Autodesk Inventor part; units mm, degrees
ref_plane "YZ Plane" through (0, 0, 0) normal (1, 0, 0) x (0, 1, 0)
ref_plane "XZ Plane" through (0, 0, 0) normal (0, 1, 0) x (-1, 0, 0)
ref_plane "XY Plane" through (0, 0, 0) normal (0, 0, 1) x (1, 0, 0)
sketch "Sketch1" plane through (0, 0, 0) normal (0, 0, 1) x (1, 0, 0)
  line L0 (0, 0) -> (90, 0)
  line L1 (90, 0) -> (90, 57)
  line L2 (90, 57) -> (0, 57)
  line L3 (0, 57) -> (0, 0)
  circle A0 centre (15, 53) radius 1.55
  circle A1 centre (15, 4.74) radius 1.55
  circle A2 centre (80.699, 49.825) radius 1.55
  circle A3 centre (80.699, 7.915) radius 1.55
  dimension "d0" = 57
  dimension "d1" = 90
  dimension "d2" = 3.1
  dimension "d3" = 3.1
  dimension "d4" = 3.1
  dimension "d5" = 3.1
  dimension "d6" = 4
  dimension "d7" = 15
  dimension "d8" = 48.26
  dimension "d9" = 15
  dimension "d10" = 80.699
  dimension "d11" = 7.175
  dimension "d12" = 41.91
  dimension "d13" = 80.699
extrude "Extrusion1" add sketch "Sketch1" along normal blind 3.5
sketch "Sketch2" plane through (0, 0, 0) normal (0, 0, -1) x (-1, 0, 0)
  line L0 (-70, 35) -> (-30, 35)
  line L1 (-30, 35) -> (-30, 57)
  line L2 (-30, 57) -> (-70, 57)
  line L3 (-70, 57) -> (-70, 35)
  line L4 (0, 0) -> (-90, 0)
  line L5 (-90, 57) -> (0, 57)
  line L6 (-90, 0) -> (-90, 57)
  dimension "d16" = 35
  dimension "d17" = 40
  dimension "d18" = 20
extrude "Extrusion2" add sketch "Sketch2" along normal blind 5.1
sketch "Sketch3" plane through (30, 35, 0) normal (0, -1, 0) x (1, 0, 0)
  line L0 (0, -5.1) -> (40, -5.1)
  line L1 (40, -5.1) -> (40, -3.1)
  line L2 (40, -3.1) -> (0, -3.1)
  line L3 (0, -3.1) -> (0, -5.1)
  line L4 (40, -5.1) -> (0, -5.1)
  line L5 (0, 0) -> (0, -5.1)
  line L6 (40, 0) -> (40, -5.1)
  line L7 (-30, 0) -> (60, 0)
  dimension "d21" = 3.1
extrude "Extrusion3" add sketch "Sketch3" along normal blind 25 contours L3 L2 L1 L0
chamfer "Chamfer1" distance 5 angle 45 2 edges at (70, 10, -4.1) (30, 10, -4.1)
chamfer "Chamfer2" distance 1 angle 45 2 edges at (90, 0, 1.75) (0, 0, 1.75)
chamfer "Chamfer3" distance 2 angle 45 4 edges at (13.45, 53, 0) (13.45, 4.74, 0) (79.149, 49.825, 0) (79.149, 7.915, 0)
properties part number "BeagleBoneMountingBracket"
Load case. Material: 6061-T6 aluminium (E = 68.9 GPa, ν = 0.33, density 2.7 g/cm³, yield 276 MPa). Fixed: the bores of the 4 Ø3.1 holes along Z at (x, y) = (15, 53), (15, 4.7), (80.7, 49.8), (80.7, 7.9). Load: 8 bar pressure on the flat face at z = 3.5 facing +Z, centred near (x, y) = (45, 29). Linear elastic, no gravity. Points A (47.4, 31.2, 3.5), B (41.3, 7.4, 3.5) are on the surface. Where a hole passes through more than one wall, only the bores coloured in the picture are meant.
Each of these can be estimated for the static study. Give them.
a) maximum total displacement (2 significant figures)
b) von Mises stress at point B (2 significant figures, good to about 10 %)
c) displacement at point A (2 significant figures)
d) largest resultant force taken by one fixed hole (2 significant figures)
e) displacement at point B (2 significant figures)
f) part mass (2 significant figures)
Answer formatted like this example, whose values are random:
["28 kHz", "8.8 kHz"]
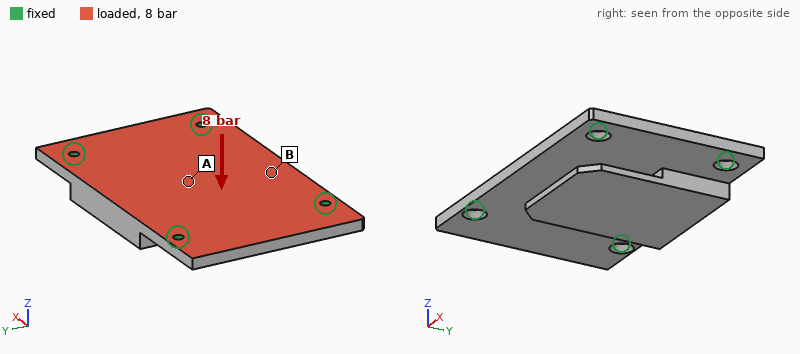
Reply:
["0.32 mm", "67 MPa", "0.19 mm", "1.8 kN", "0.22 mm", "65 g"]
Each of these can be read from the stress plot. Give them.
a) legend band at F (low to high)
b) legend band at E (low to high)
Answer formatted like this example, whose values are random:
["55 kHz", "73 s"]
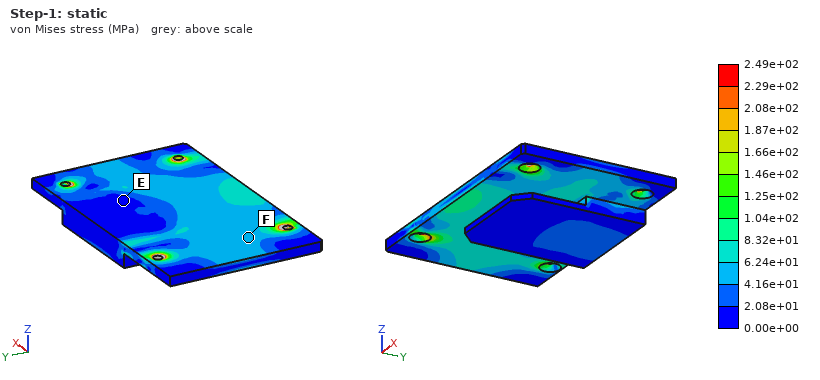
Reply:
["4.16e+01 to 6.24e+01 MPa", "0.00e+00 to 2.08e+01 MPa"]
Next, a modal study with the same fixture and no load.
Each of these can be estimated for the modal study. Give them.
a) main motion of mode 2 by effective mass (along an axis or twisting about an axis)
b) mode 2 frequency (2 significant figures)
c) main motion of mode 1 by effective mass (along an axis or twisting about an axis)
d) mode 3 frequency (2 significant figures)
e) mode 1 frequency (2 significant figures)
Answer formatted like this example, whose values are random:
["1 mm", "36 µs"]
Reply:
["along Z", "3600 Hz", "along Z", "4600 Hz", "2200 Hz"]
